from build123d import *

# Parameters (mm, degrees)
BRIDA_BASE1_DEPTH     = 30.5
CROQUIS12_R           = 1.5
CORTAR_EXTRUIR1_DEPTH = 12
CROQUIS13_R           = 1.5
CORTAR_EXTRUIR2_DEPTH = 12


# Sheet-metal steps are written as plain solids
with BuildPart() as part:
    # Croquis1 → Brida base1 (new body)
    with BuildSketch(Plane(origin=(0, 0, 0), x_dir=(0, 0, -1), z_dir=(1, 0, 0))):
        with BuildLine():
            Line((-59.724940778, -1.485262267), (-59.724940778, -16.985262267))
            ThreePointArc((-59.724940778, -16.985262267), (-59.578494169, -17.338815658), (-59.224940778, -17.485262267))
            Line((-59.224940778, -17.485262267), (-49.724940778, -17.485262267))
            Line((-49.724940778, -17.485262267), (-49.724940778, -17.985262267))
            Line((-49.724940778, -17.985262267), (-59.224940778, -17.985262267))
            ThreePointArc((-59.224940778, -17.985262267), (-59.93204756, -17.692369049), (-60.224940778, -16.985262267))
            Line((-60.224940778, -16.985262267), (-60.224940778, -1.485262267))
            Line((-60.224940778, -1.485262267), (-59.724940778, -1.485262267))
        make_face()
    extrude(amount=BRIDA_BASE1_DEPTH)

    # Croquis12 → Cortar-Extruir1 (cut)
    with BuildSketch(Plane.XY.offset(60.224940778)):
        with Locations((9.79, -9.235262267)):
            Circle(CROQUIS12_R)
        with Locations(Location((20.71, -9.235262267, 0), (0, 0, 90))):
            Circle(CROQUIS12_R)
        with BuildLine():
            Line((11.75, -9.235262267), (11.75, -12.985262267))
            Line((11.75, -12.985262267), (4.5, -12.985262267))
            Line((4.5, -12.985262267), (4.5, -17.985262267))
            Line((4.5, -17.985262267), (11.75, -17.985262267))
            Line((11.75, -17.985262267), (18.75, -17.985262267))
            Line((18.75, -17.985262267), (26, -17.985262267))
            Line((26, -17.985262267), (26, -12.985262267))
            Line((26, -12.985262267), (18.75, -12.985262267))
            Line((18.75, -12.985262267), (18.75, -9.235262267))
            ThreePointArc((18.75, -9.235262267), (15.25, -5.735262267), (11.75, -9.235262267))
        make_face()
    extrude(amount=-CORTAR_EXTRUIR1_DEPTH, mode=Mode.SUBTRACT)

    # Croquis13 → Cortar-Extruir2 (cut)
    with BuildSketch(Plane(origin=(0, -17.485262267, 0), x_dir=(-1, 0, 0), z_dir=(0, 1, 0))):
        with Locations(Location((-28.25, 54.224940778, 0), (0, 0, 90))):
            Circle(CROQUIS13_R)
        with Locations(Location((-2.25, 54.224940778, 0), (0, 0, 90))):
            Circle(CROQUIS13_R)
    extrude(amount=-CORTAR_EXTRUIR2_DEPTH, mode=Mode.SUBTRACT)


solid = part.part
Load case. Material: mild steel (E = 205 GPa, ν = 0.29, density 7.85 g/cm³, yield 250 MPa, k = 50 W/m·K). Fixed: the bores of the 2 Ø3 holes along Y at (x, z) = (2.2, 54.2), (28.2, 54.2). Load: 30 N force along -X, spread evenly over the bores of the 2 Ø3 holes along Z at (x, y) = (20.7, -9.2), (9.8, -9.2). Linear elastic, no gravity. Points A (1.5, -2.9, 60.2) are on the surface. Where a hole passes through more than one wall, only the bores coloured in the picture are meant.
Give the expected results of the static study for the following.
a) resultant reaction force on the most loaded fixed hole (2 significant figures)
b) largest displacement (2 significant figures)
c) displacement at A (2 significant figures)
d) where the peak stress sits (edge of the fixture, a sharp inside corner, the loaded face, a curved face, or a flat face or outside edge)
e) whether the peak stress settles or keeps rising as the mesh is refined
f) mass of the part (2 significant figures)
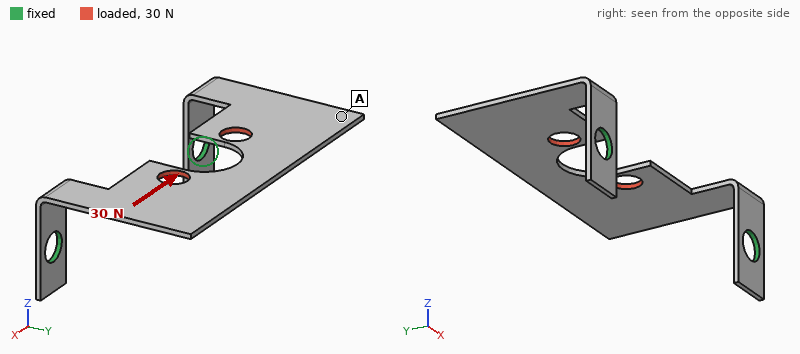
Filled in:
18 N
68 µm
60 µm
edge of the fixture
keeps rising
1.6 g
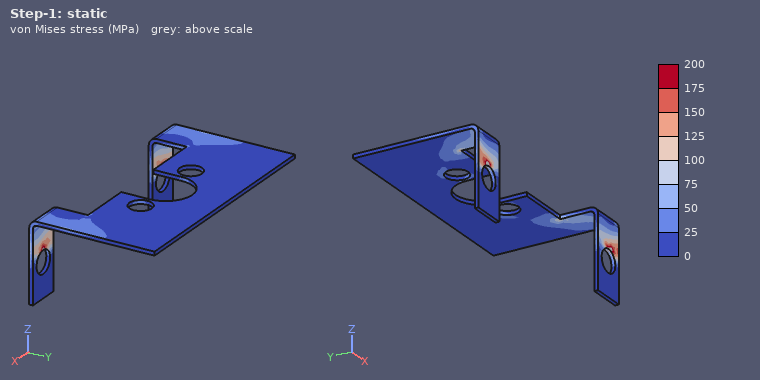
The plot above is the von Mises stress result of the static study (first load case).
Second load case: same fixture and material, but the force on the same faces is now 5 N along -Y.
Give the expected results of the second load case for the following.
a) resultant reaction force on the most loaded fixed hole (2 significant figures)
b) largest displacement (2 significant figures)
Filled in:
2.7 N
41 µm
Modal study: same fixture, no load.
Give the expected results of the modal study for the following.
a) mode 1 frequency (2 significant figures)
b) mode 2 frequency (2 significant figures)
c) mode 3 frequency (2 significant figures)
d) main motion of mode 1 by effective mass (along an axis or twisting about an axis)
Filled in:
630 Hz
1600 Hz
3500 Hz
along Z
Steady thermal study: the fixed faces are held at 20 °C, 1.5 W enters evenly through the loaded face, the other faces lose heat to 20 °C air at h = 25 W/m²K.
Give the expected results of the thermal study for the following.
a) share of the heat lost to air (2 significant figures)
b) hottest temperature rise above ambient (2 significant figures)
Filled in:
51 %
62 K
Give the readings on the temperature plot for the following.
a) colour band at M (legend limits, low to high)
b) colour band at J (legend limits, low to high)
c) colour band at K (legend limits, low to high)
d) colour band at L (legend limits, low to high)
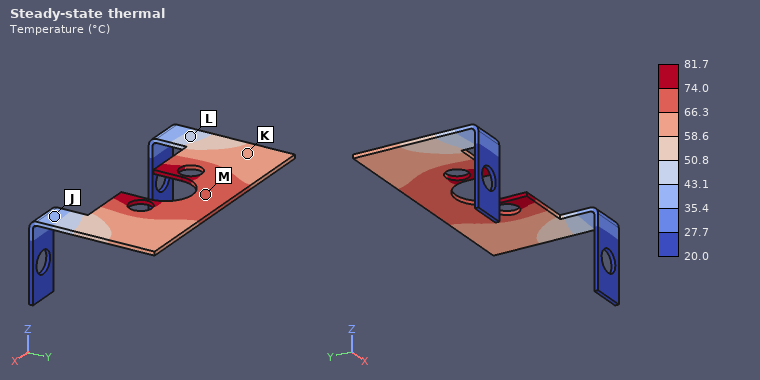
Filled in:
66.3 to 74.0 °C
35.4 to 43.1 °C
58.6 to 66.3 °C
43.1 to 50.8 °C
